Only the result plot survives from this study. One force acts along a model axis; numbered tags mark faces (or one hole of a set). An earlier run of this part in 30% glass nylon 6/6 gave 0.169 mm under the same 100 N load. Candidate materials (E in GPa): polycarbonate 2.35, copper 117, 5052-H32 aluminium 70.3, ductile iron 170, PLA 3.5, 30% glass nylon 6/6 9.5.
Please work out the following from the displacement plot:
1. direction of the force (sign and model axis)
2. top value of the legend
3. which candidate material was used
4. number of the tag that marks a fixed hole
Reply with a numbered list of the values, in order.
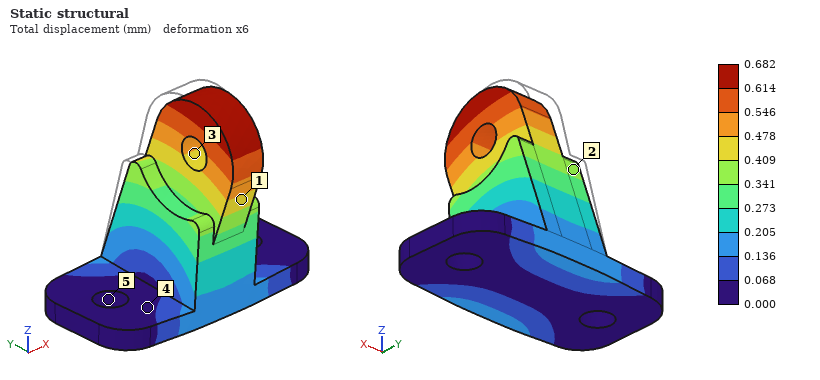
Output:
1. -Y
2. 0.682 mm
3. polycarbonate
4. 5
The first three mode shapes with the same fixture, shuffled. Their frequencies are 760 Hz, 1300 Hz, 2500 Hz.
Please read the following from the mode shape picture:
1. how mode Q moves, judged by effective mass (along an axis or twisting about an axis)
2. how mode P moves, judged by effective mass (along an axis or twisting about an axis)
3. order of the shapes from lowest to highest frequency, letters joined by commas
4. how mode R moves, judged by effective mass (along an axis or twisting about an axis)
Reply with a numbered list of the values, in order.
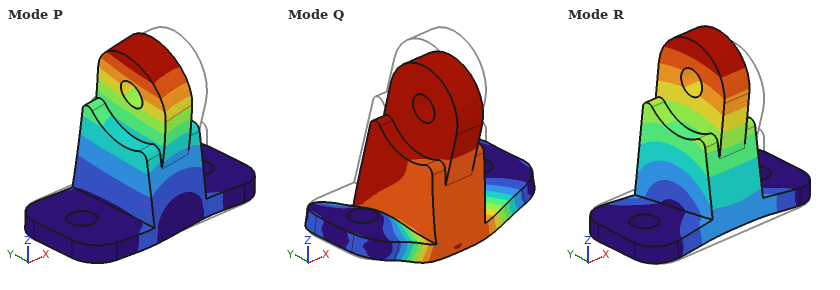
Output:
1. along Z
2. along X
3. R, P, Q
4. along Y
